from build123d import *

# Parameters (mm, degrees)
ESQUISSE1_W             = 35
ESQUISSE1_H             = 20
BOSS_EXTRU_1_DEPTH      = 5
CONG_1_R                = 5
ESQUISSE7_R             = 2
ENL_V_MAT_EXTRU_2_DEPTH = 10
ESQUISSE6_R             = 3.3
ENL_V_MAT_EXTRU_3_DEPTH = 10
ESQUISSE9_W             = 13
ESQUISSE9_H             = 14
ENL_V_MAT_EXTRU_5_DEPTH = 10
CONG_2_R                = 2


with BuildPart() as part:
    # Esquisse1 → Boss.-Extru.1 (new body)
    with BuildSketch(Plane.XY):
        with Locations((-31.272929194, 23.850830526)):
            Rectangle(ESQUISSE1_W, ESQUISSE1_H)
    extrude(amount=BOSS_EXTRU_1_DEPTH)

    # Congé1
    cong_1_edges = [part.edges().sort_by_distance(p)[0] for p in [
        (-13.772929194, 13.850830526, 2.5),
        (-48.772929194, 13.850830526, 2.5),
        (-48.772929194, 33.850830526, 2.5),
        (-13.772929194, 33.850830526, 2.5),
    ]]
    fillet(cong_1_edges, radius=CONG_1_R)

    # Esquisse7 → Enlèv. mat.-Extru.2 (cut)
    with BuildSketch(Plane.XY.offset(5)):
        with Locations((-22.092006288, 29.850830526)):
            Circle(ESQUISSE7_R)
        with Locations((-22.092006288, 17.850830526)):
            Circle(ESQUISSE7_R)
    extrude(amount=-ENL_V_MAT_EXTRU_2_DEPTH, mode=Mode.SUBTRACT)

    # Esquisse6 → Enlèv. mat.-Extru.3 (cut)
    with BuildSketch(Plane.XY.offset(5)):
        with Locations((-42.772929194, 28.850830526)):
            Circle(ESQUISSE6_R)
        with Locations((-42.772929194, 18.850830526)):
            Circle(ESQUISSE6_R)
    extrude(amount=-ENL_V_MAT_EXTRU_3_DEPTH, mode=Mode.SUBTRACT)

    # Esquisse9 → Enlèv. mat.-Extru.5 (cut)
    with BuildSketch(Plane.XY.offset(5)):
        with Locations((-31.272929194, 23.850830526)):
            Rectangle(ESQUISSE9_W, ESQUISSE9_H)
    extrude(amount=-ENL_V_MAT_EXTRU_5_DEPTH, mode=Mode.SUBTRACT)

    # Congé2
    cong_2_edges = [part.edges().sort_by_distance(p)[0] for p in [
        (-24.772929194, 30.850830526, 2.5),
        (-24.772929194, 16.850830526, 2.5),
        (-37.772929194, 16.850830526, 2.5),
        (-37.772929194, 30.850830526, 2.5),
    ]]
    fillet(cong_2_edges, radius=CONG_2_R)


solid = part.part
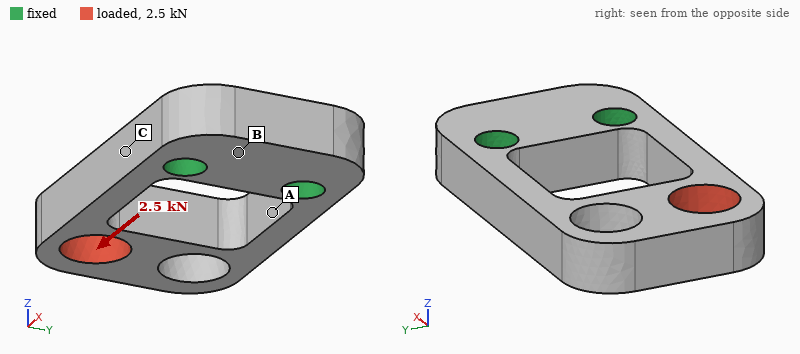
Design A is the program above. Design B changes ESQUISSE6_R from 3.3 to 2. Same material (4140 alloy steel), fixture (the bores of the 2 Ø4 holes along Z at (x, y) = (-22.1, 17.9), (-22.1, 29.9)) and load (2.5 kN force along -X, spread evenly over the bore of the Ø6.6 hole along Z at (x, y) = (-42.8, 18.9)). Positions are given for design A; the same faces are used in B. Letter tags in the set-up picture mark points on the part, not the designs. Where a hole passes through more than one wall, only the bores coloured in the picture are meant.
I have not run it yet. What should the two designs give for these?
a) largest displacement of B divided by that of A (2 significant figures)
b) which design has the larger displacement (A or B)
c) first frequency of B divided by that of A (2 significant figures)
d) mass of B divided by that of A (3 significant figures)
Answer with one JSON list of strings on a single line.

["0.71", "A", "0.90", "1.11"]
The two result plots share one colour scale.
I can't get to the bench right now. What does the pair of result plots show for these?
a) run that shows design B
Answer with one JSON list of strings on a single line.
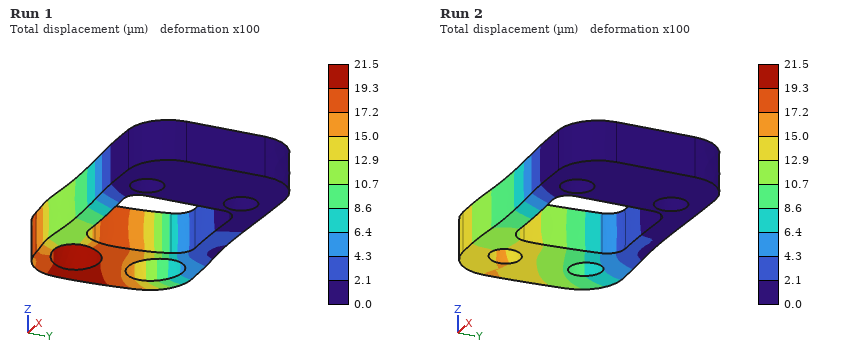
["Run 2"]
